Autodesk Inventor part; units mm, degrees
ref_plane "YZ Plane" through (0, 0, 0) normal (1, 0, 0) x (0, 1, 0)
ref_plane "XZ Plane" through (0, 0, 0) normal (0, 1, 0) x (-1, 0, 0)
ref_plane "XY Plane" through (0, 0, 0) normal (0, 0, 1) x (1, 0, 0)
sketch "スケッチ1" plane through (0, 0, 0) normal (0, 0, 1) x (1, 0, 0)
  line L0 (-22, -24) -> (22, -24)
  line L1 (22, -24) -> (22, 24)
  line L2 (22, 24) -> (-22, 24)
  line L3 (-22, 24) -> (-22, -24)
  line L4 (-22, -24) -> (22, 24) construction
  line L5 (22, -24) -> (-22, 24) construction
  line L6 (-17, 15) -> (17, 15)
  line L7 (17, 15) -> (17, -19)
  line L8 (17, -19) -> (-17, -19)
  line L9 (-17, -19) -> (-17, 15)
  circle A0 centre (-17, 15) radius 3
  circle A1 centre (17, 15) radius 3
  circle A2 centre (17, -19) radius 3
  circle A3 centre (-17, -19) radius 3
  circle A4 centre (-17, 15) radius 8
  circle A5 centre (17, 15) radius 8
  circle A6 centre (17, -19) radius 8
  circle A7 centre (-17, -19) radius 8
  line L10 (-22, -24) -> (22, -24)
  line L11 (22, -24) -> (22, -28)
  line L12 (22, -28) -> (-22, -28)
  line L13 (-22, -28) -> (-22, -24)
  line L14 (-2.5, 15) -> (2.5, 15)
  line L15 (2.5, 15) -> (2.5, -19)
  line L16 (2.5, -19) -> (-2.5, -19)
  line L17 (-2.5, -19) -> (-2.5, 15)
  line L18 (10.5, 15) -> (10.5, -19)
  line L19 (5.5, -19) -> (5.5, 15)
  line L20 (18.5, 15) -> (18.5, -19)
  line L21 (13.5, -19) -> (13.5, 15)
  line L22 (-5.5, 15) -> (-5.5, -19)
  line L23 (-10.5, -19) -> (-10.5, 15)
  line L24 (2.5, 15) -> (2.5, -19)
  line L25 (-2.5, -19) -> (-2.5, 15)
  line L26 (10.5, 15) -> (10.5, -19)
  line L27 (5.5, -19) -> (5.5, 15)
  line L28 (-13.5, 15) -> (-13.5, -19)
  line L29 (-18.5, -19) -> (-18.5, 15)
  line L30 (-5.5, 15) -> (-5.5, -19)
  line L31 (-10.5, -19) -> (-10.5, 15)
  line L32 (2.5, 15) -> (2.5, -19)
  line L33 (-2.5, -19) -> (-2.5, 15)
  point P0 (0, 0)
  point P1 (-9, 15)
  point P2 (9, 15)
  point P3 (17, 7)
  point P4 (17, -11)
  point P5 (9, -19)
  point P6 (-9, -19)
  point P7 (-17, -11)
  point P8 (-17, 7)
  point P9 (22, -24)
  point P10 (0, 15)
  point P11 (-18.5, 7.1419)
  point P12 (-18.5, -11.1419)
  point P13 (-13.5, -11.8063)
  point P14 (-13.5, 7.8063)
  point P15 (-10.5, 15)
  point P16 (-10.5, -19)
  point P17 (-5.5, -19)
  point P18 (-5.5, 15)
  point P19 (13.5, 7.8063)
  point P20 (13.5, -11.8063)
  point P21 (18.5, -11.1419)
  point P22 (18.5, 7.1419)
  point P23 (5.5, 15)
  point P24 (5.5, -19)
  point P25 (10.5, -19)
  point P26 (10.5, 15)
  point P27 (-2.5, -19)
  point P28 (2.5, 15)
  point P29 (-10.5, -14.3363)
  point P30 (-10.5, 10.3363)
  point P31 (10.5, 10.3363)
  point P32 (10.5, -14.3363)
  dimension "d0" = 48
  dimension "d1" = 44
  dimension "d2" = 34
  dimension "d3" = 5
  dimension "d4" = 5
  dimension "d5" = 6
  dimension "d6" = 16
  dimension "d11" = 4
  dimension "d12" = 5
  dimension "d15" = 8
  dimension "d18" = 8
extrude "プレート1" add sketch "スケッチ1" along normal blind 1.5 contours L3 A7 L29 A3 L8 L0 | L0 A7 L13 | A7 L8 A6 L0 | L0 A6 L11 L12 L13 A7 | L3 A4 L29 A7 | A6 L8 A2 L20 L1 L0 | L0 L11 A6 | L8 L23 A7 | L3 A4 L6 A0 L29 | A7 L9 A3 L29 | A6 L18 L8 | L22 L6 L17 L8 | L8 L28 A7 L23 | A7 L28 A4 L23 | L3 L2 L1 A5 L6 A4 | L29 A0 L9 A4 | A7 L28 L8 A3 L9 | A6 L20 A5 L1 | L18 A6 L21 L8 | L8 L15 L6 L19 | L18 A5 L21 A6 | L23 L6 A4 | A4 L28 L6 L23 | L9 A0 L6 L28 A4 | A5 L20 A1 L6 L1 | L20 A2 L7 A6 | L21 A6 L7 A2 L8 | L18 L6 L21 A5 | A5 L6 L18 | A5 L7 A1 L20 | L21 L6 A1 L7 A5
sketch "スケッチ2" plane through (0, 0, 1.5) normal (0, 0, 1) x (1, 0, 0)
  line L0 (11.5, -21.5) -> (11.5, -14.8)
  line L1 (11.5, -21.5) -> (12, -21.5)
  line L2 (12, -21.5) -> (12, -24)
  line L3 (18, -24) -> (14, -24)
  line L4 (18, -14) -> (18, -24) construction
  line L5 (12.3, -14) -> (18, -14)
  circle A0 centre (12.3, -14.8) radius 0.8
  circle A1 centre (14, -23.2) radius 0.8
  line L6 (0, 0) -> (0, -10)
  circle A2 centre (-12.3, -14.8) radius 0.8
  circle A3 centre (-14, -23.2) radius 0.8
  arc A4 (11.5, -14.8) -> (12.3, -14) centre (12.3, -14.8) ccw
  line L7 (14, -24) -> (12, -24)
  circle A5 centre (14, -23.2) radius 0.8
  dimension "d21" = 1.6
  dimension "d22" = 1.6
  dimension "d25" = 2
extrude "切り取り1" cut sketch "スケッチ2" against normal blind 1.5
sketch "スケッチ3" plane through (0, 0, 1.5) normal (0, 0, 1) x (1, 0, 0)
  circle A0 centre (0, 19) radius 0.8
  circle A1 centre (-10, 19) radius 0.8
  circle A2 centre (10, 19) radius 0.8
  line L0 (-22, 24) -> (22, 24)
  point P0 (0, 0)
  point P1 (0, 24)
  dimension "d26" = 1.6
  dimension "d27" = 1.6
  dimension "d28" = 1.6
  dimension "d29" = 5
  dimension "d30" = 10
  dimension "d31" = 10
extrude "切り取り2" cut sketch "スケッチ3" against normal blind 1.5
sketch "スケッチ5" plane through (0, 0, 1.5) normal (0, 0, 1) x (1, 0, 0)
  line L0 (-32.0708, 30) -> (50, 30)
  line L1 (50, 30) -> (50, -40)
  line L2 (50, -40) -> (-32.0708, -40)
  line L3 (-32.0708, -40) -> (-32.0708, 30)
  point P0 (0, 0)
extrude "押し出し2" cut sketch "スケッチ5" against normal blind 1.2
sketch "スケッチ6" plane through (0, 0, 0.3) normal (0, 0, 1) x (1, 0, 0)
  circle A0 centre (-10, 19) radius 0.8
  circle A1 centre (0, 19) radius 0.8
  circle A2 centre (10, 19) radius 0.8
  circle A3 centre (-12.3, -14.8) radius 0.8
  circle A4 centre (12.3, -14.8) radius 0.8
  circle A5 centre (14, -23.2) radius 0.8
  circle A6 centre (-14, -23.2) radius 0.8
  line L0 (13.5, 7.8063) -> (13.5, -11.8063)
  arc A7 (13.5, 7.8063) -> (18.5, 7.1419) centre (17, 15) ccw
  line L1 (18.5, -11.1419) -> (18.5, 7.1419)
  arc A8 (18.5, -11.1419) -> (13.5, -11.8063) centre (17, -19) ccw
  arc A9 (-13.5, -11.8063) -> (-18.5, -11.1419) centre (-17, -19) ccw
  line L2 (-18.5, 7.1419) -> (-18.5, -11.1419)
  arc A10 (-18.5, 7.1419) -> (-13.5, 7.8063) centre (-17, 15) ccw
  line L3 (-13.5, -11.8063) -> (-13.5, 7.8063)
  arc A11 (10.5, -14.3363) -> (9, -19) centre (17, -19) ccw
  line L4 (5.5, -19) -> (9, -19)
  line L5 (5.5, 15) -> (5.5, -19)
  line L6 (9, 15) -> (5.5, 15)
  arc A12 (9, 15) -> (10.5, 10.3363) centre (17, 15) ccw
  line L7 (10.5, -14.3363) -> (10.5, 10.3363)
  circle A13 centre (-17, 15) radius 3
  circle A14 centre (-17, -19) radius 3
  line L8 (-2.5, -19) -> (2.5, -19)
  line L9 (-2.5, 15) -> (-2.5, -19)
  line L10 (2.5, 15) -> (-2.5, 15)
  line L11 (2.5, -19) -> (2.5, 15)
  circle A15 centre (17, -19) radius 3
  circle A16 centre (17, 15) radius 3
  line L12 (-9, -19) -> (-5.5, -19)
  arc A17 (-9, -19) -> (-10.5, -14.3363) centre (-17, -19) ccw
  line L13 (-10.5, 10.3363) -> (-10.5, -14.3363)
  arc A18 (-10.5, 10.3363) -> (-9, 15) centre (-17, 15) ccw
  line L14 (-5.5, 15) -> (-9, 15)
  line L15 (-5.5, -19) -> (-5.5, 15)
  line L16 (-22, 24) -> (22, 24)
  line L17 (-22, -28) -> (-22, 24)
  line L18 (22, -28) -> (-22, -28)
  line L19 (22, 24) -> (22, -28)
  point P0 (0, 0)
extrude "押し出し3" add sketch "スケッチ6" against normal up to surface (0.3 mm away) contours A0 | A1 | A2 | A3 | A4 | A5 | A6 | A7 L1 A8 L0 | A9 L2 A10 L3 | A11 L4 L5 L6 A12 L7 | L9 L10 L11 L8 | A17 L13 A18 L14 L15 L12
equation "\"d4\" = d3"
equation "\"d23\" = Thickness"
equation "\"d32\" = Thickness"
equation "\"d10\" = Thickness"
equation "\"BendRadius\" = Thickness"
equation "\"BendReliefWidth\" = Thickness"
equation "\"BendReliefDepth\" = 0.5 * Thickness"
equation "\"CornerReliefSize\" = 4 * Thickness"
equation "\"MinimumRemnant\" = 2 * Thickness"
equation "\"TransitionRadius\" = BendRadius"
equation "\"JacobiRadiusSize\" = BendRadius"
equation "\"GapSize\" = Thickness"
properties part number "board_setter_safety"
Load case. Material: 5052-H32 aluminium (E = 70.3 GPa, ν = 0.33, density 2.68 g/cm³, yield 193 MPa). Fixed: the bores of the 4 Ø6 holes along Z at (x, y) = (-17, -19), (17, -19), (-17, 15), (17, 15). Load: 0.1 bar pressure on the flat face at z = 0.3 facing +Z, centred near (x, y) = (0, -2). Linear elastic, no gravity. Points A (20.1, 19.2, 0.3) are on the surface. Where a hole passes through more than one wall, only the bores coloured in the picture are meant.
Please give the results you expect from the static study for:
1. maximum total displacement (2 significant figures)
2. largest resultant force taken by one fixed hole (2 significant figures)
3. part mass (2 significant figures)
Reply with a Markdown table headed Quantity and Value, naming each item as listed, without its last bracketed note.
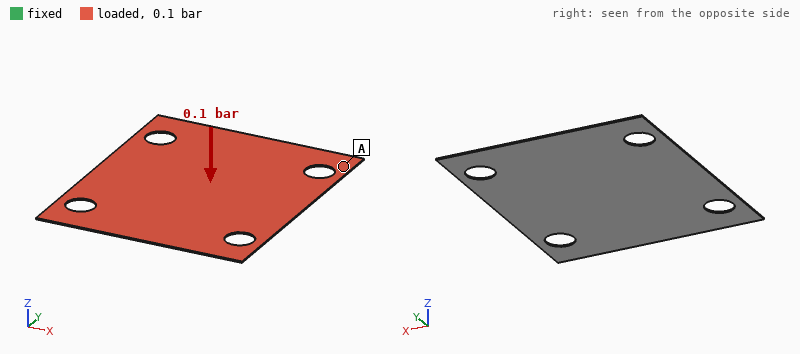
| Quantity | Value |
|---|---|
| maximum total displacement | 0.30 mm |
| largest resultant force taken by one fixed hole | 5.5 N |
| part mass | 1.7 g |
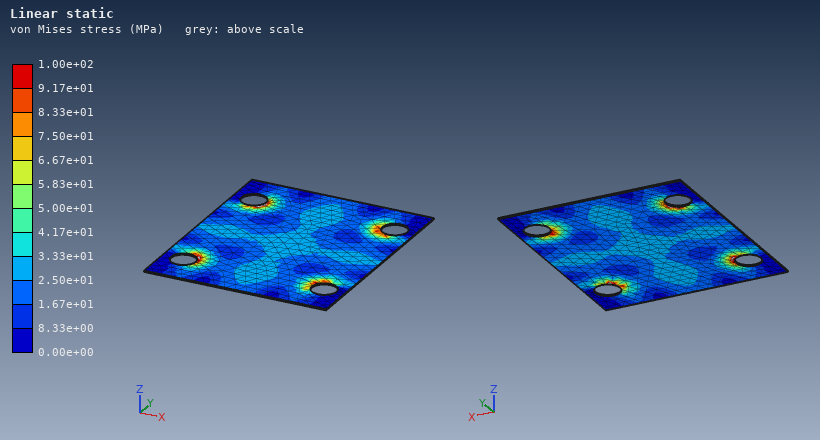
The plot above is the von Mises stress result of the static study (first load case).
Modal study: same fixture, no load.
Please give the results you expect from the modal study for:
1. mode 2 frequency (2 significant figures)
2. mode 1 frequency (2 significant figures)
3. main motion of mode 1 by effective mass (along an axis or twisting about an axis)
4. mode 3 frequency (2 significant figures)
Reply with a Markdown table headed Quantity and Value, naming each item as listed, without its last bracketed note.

| Quantity | Value |
|---|---|
| mode 2 frequency | 1800 Hz |
| mode 1 frequency | 1300 Hz |
| main motion of mode 1 by effective mass | along Z |
| mode 3 frequency | 1900 Hz |
